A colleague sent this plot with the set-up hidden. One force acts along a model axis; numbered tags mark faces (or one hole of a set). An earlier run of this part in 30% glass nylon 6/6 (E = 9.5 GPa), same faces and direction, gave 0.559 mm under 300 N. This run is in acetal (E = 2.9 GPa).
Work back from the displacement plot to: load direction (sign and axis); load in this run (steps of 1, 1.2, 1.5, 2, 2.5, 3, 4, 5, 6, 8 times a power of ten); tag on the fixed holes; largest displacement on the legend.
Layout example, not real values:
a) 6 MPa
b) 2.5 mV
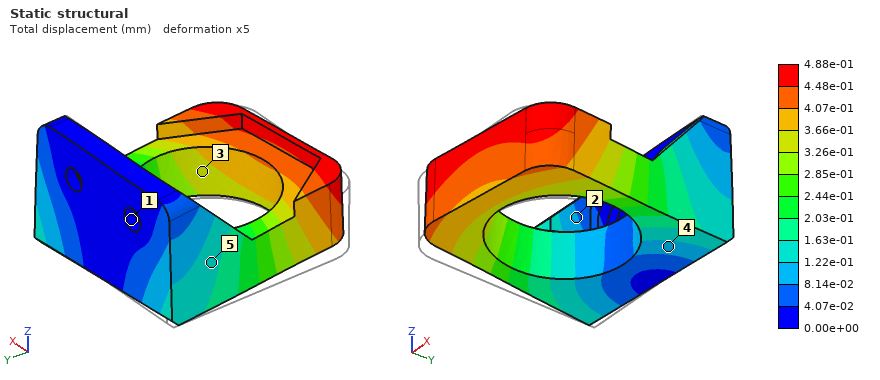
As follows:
a) +X
b) 80 N
c) 1
d) 4.88e-01 mm
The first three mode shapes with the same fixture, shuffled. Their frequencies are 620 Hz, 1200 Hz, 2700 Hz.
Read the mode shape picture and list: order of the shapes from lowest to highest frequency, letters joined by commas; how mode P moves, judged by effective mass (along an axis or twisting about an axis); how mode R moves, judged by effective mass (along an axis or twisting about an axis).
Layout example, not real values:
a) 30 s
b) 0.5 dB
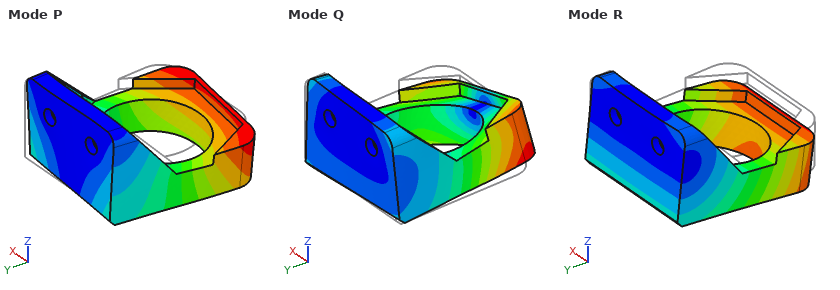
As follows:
a) R, P, Q
b) along X
c) along Z
